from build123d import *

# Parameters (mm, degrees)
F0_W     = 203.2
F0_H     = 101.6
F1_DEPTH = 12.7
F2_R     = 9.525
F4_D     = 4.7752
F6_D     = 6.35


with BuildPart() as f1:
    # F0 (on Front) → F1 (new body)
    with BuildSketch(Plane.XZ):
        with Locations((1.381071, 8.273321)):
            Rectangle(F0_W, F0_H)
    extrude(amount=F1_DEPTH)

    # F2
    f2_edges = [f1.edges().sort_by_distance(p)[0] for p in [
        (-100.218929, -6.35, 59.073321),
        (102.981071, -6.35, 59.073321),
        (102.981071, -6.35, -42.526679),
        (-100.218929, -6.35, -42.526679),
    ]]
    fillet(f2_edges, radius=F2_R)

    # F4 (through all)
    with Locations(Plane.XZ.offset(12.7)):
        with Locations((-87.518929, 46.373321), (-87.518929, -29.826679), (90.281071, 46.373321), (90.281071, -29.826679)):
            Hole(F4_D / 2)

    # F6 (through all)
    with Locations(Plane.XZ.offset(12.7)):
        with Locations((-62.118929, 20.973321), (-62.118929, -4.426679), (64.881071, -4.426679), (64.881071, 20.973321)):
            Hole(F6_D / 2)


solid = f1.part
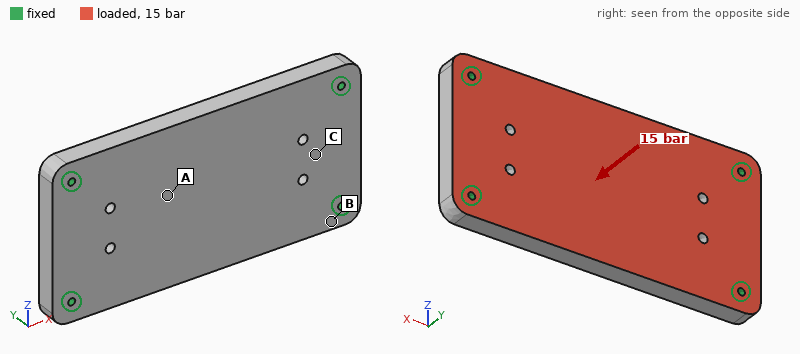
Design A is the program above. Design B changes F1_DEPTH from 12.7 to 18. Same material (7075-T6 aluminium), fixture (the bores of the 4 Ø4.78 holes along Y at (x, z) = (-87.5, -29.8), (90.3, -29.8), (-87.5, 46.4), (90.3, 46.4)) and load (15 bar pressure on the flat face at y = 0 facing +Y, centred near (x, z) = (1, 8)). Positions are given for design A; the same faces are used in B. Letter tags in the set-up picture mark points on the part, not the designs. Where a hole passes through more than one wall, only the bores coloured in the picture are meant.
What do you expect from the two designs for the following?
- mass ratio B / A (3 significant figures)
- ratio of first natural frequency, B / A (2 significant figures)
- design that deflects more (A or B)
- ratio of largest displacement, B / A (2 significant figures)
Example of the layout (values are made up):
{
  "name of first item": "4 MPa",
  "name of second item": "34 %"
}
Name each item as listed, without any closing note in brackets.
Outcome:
{
  "mass ratio B / A": "1.42",
  "ratio of first natural frequency, B / A": "1.3",
  "design that deflects more": "A",
  "ratio of largest displacement, B / A": "0.39"
}
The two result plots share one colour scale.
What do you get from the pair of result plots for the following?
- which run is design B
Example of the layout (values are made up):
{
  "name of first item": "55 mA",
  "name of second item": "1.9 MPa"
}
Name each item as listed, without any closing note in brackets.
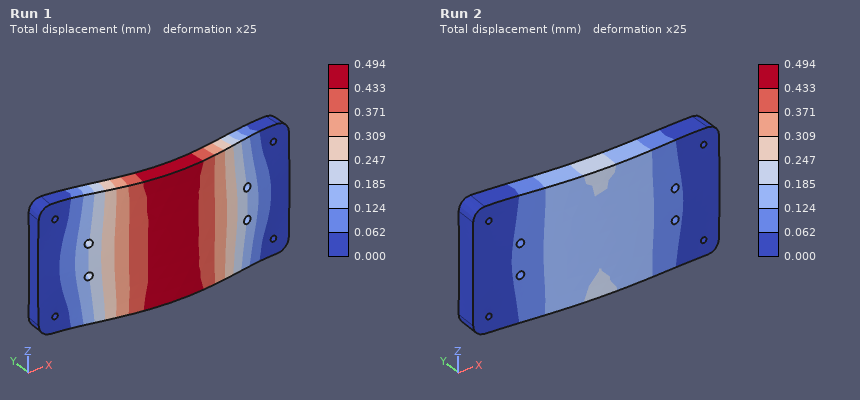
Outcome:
{
  "which run is design B": "Run 2"
}
